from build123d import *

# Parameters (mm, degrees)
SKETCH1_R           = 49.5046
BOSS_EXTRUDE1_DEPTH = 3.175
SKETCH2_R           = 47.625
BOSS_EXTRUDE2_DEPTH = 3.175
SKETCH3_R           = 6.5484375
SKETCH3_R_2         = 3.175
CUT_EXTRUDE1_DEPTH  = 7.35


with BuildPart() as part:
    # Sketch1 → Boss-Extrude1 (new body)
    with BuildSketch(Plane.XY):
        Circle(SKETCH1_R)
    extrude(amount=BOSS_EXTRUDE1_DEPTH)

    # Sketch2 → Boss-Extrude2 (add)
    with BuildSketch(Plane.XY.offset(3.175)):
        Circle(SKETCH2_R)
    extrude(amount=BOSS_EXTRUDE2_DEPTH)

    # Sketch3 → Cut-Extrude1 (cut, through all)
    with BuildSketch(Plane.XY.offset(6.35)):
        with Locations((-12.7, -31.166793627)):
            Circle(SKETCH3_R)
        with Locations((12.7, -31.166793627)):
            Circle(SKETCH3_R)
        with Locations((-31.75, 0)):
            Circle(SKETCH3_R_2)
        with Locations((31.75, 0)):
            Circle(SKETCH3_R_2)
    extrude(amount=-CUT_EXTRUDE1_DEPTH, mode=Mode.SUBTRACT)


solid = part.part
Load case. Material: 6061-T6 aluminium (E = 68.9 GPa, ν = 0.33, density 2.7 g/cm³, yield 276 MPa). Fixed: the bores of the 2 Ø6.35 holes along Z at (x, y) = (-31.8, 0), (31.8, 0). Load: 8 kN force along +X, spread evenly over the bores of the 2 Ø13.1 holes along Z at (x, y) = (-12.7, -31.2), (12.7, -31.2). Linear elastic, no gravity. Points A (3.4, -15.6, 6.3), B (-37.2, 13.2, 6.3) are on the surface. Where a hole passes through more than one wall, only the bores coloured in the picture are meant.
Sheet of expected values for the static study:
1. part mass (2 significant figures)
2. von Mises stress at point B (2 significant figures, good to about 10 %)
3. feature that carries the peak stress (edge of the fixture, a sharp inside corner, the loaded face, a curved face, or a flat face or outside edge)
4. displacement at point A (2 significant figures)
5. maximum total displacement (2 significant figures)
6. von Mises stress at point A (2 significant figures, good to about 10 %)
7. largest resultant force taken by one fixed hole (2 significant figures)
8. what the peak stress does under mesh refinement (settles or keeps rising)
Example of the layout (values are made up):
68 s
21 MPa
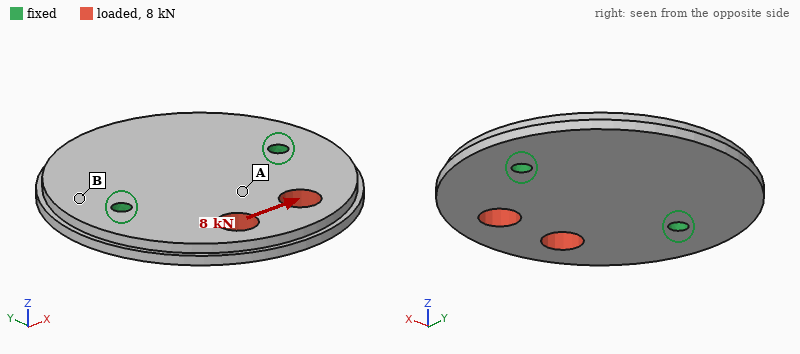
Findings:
120 g
11 MPa
edge of the fixture
14 µm
37 µm
26 MPa
5.4 kN
keeps rising
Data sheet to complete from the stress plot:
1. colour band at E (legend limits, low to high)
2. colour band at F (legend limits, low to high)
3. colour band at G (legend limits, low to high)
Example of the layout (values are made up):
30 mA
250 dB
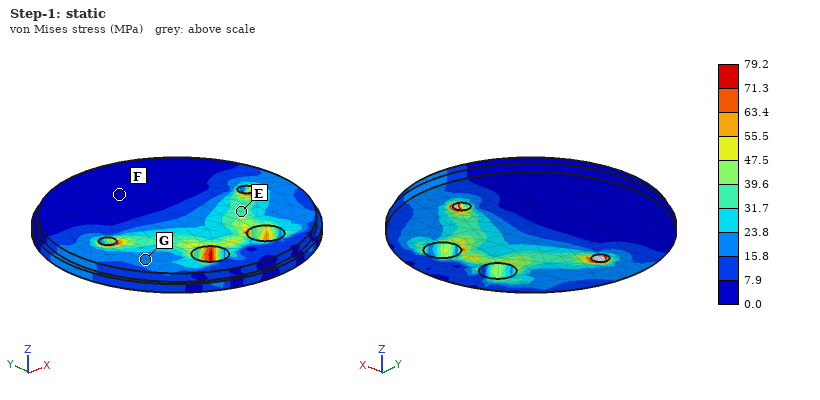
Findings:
31.7 to 39.6 MPa
0.0 to 7.9 MPa
15.8 to 23.8 MPa
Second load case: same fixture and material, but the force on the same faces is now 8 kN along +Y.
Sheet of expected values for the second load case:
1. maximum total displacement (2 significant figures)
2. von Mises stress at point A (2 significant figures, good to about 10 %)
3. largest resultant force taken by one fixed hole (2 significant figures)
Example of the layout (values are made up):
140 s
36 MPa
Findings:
19 µm
17 MPa
4.1 kN
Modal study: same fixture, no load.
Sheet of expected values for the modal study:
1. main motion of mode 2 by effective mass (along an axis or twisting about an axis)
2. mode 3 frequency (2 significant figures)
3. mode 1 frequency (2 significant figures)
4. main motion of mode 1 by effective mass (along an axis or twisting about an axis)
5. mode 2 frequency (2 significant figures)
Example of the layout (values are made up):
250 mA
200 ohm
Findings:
along Z
5300 Hz
2200 Hz
twisting about X
2800 Hz
